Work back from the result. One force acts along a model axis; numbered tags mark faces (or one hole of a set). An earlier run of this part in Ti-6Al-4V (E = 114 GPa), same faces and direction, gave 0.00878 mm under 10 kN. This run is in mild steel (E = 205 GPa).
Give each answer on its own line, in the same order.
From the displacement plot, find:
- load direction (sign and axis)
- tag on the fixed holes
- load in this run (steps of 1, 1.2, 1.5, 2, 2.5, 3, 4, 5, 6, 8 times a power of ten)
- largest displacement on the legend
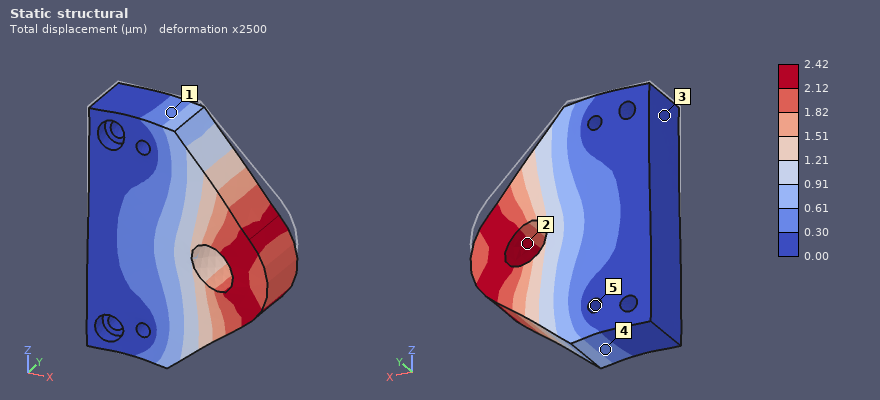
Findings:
-Z
5
5 kN
2.42 µm
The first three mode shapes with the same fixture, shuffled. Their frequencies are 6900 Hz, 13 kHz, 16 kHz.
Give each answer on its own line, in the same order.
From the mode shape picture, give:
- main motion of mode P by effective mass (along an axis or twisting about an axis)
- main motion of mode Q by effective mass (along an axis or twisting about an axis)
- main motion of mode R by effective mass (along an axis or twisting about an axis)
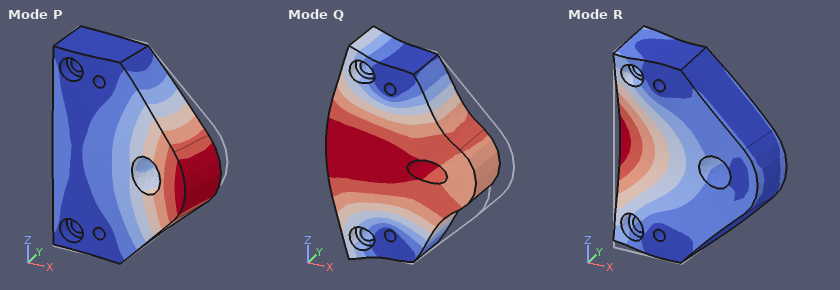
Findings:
along Y
along X
along Y
